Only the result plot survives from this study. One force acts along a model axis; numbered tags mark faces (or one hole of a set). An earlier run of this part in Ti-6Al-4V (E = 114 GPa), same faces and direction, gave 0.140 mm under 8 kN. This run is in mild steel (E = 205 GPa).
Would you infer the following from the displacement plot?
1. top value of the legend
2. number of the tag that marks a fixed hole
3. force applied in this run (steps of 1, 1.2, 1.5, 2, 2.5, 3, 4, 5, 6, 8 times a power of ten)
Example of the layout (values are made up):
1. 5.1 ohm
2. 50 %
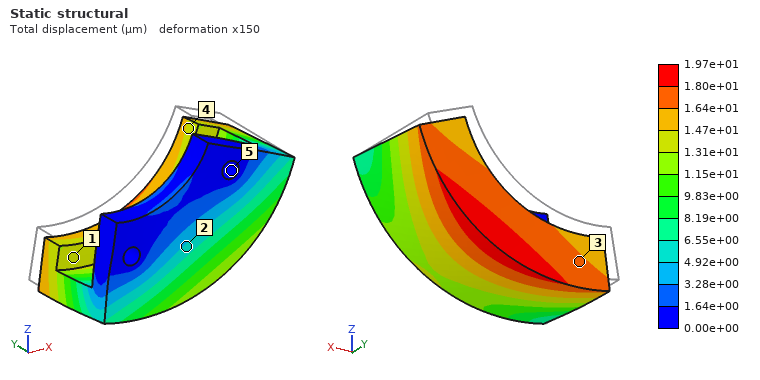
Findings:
1. 1.97e+01 µm
2. 5
3. 2 kN
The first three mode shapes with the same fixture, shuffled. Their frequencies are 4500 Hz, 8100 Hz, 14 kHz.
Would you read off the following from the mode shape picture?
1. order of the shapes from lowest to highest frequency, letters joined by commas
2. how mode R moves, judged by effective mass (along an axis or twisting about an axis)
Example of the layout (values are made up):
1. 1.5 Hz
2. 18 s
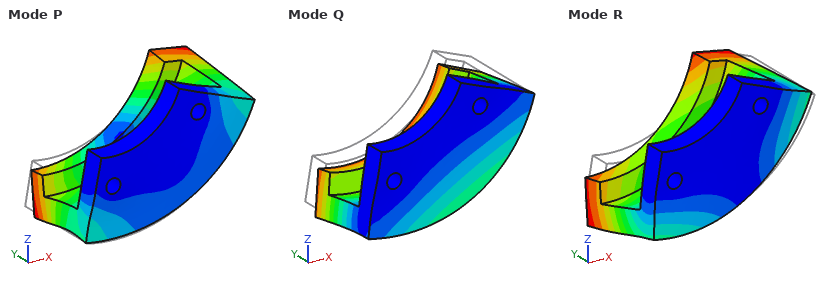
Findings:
1. Q, R, P
2. along X
